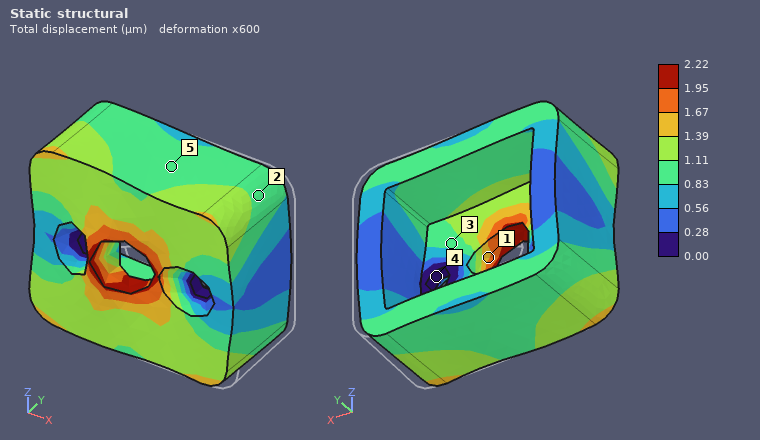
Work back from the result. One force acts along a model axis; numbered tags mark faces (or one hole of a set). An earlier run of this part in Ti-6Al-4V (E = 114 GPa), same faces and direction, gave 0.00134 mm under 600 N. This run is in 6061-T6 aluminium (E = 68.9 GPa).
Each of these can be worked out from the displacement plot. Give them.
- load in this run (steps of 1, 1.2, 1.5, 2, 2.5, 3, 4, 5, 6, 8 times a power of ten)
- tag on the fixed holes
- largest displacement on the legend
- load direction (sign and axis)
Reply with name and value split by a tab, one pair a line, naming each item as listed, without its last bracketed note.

load in this run	600 N
tag on the fixed holes	4
largest displacement on the legend	2.22 µm
load direction	-X
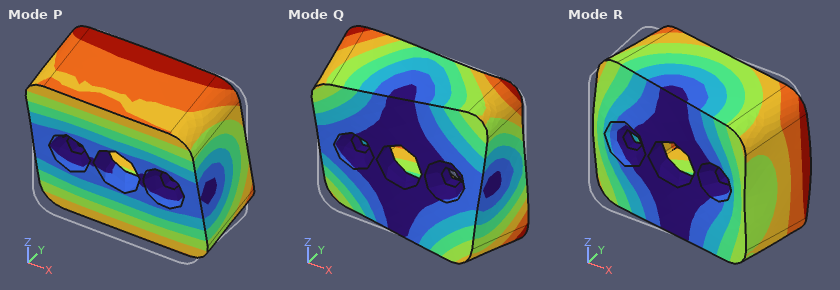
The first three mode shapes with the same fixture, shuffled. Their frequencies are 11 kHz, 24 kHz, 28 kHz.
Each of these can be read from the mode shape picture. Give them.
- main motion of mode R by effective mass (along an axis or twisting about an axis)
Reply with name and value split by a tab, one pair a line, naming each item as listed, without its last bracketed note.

main motion of mode R by effective mass	along X
